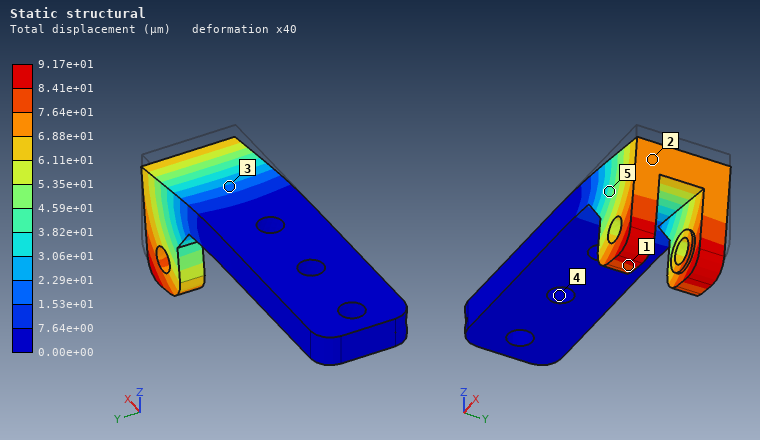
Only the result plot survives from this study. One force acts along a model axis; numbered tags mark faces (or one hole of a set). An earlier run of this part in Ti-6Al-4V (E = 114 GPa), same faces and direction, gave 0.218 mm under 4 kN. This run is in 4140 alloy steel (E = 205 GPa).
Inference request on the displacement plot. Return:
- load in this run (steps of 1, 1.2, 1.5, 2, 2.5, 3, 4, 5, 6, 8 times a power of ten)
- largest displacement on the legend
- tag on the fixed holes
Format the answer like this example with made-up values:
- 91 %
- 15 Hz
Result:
- 3 kN
- 9.17e+01 µm
- 4
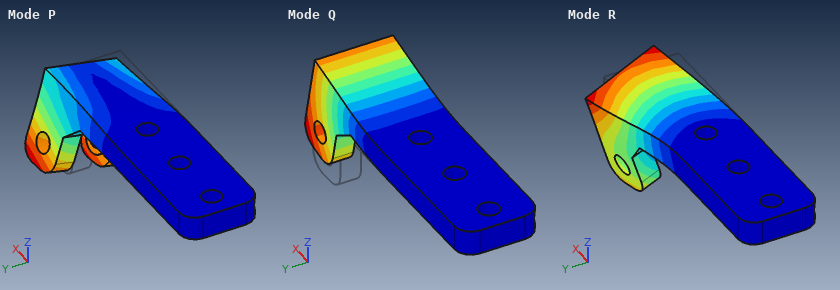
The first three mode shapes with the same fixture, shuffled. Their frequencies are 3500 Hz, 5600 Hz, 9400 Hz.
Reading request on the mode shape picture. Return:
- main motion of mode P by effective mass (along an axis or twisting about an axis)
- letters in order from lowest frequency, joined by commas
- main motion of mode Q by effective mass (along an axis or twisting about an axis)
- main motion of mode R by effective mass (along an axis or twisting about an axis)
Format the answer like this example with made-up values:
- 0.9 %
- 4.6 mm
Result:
- along Y
- Q, P, R
- along Z
- along Y
